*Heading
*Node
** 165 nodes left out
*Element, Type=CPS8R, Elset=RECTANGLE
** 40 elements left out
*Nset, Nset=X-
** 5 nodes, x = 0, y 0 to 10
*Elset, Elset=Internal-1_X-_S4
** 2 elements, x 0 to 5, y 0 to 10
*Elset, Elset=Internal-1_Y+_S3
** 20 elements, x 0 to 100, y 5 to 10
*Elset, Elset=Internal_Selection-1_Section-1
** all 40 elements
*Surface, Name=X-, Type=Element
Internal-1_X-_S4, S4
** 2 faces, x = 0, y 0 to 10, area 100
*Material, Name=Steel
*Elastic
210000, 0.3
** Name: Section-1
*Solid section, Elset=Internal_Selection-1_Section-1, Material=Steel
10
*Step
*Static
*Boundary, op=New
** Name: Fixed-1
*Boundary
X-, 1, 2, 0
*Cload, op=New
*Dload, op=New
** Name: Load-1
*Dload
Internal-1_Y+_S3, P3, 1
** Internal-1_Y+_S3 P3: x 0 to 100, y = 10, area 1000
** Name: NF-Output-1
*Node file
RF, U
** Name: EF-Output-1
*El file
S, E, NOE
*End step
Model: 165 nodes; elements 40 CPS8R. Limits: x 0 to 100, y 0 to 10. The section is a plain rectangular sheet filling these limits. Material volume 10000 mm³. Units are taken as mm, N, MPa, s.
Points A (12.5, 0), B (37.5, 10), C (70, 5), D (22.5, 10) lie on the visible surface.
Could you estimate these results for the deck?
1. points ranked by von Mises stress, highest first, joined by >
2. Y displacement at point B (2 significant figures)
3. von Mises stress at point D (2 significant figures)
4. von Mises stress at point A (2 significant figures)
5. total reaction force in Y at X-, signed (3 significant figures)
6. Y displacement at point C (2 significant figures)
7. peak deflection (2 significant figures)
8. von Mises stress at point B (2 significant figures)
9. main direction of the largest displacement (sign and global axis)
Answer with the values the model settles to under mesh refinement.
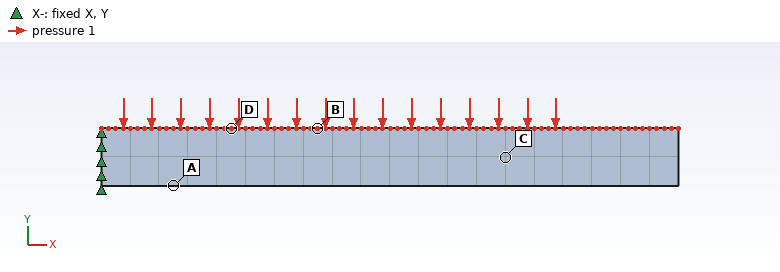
A > D > B > C
-0.16 mm
170 MPa
220 MPa
1000 N
-0.43 mm
0.71 mm
110 MPa
-Y
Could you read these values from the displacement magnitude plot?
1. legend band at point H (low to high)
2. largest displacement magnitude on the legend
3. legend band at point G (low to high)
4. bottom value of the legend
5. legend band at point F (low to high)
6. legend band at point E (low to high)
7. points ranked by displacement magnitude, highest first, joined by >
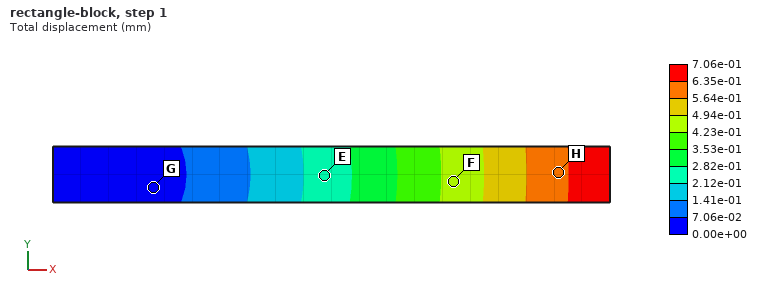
5.64e-01 to 6.35e-01 mm
7.06e-01 mm
0.00e+00 to 7.06e-02 mm
0.00e+00 mm
4.23e-01 to 4.94e-01 mm
2.12e-01 to 2.82e-01 mm
H > F > E > G
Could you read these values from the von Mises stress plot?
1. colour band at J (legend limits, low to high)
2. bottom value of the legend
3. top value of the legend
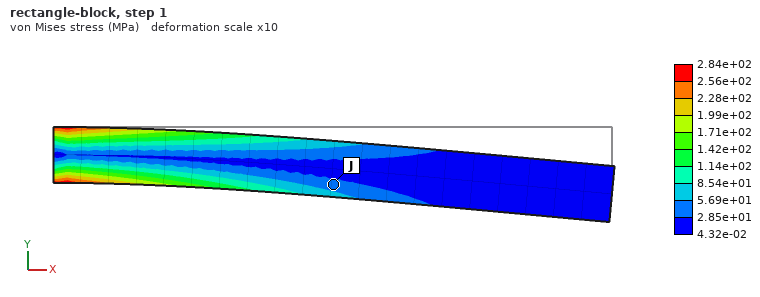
2.85e+01 to 5.69e+01 MPa
4.32e-02 MPa
2.84e+02 MPa
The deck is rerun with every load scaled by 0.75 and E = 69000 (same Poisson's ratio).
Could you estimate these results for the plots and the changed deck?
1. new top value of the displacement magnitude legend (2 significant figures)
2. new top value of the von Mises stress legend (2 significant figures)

1.6 mm
210 MPa
